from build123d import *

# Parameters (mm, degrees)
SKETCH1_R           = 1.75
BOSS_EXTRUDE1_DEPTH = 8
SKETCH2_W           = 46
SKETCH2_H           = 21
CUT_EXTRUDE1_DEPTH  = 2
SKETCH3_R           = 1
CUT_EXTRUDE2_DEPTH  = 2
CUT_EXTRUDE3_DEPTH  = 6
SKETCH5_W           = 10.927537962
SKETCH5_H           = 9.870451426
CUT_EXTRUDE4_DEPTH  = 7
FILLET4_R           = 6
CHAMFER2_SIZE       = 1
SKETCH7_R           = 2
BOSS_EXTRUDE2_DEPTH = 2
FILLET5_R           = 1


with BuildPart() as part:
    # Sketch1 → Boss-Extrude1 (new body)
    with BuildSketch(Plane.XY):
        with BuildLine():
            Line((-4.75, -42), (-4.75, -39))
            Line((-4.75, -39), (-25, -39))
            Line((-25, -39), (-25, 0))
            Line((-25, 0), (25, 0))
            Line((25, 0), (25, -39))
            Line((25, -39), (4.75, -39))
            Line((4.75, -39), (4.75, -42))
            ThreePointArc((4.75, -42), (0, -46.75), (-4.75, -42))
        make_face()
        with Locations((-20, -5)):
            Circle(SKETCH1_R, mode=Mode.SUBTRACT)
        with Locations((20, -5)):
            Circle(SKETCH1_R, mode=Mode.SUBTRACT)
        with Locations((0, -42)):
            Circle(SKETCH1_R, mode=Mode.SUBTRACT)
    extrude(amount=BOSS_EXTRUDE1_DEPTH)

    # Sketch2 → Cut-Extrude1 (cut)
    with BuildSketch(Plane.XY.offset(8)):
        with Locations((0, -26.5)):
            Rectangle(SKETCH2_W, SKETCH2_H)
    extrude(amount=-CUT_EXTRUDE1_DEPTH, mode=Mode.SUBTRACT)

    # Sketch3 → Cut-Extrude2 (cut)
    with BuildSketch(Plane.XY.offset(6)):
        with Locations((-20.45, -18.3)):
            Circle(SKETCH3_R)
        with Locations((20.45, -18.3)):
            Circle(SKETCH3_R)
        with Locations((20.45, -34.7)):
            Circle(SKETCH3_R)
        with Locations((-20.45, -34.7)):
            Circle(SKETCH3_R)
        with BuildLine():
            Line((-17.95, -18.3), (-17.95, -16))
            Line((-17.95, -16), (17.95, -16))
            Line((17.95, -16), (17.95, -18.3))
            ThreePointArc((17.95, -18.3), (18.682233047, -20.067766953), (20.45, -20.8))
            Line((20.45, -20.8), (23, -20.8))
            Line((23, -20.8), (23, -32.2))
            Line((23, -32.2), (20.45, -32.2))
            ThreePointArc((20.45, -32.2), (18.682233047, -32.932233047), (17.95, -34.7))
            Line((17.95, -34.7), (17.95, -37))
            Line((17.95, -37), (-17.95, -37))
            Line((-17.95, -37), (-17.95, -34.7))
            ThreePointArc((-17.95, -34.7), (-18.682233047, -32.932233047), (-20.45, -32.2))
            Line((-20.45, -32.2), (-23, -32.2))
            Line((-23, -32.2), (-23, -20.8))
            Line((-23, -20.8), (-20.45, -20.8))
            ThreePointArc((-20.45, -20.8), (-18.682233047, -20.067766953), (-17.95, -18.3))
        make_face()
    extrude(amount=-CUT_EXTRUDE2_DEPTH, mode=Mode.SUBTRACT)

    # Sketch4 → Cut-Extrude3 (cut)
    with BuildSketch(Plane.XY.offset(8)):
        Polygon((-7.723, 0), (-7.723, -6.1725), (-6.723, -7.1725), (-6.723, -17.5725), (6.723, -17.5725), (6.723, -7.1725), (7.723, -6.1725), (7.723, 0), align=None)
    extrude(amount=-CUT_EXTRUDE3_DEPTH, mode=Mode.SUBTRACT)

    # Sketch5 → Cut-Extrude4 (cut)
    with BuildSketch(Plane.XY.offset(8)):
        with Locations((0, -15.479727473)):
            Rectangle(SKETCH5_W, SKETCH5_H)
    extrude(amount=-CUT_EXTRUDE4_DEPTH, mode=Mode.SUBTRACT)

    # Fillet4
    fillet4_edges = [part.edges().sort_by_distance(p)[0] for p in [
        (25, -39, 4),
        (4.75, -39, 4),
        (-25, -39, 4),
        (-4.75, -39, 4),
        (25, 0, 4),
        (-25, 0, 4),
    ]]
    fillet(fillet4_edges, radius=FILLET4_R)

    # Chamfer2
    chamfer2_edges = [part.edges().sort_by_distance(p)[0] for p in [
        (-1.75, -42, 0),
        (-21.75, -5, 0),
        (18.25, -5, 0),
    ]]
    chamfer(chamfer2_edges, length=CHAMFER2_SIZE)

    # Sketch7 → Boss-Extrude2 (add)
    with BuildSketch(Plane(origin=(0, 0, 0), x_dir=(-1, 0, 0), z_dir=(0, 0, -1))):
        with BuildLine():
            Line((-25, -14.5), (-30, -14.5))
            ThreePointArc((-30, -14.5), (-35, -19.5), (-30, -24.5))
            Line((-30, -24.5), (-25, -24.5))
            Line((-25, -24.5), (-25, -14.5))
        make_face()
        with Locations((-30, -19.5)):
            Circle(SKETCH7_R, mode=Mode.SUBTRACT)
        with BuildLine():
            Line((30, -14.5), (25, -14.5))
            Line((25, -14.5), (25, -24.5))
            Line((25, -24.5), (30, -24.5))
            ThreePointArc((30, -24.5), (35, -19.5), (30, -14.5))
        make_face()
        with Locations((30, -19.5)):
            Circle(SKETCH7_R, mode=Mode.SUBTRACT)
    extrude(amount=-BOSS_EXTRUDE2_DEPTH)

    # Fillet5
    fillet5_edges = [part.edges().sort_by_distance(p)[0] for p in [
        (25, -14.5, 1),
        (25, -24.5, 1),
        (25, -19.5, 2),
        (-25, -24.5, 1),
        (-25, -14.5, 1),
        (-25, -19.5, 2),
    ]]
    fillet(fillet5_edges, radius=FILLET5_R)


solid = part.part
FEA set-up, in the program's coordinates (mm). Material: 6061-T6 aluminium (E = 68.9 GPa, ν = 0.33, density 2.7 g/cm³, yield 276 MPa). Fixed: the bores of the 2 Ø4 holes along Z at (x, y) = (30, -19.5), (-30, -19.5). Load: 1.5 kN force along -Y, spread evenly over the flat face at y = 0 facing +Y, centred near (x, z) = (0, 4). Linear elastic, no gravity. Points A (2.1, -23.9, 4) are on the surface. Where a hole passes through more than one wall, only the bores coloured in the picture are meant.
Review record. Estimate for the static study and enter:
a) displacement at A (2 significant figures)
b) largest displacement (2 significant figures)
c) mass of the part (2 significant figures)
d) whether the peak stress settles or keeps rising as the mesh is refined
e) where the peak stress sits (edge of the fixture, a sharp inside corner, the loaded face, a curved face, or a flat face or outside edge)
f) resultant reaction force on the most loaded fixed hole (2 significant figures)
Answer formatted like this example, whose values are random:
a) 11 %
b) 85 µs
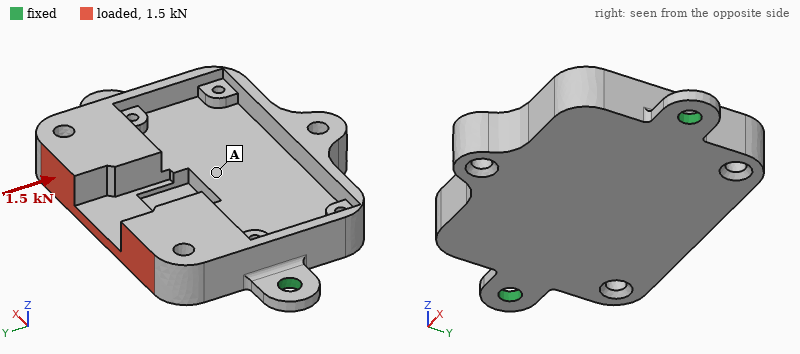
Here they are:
a) 0.054 mm
b) 0.22 mm
c) 29 g
d) keeps rising
e) edge of the fixture
f) 750 N
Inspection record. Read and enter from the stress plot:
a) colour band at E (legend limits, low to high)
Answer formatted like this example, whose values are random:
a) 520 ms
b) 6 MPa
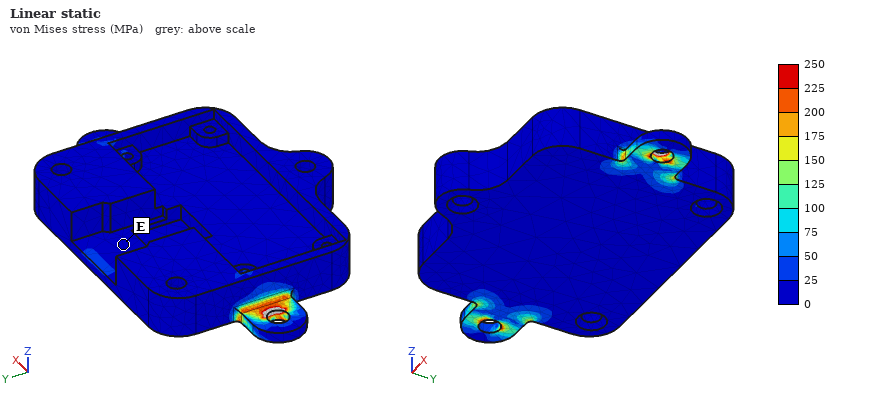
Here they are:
a) 0 to 25 MPa
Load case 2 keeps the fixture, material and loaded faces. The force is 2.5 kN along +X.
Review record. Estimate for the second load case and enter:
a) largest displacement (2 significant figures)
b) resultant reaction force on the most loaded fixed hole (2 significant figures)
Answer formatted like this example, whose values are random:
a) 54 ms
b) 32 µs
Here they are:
a) 31 µm
b) 1.5 kN
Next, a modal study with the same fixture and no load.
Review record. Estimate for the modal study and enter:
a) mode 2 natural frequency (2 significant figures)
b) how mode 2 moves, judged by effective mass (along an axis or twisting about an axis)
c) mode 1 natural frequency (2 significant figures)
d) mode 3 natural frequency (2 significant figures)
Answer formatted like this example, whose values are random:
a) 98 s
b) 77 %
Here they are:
a) 2900 Hz
b) along Z
c) 1700 Hz
d) 5400 Hz
